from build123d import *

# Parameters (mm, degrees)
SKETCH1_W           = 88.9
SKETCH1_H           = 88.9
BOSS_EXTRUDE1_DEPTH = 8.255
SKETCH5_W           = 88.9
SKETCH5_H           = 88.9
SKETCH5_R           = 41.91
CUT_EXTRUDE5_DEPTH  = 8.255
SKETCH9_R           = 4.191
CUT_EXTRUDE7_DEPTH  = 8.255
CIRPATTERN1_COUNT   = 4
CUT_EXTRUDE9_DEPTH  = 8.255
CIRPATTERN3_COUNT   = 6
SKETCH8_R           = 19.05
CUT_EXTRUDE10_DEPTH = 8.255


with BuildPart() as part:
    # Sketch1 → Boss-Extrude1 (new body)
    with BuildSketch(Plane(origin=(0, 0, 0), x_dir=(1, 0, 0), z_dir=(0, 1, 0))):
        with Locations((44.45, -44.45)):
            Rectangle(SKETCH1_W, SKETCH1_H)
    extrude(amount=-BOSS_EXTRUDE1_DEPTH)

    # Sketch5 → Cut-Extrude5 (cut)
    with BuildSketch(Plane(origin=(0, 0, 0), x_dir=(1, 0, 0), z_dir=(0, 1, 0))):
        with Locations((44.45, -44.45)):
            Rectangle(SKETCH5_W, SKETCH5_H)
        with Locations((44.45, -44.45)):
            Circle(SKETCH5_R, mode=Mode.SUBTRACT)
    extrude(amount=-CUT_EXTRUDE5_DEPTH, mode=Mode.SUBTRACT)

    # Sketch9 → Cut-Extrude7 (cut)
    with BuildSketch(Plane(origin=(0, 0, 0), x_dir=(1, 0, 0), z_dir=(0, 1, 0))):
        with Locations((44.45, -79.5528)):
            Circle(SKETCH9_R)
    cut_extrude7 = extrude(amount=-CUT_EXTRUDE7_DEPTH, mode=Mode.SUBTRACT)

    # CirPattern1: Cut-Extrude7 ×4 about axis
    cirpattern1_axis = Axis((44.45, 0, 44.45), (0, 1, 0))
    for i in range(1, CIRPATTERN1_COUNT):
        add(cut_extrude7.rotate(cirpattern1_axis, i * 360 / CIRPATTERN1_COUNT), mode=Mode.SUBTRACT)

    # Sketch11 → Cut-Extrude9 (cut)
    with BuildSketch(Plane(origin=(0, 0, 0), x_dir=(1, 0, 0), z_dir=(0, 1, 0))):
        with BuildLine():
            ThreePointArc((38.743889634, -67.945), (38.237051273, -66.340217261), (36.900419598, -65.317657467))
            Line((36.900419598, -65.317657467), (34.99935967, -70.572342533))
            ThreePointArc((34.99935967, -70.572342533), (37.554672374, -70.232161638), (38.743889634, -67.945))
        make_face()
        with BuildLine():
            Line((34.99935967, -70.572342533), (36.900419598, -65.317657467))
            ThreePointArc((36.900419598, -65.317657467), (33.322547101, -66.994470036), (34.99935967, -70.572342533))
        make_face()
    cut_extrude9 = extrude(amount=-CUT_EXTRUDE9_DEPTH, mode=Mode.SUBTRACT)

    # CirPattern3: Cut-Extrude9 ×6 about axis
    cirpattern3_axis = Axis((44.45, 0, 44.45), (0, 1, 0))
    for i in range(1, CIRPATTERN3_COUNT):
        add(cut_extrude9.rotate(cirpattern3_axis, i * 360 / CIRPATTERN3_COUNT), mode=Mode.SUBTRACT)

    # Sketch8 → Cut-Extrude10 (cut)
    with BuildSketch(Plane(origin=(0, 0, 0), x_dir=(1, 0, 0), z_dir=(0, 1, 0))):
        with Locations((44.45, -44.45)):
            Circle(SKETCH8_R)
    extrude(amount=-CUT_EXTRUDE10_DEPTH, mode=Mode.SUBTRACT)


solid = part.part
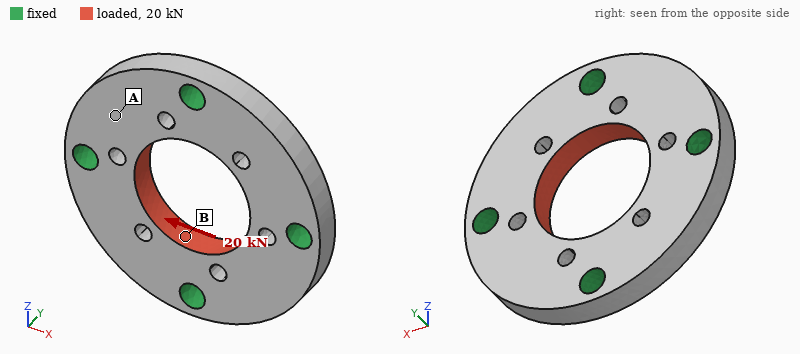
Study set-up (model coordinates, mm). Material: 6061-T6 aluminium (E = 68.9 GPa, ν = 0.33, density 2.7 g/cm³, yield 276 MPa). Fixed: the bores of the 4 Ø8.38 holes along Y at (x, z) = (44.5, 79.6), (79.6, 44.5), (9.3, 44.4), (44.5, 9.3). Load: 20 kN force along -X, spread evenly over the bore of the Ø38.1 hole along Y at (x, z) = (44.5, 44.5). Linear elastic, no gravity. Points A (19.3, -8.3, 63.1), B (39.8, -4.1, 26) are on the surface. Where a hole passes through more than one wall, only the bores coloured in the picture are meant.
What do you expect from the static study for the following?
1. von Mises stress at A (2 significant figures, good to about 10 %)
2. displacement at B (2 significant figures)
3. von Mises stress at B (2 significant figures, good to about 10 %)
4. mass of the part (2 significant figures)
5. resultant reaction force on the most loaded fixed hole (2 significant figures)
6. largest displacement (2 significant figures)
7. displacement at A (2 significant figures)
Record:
10.0 MPa
14 µm
35 MPa
89 g
5.3 kN
15 µm
10 µm
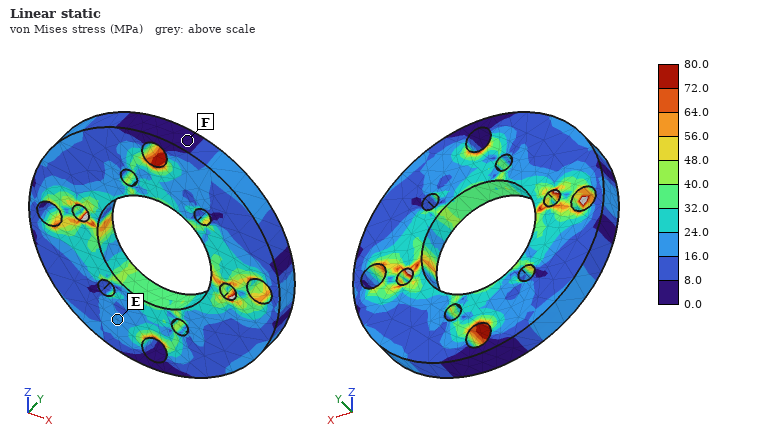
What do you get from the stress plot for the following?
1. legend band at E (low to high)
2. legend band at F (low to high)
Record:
16.0 to 24.0 MPa
0.0 to 8.0 MPa
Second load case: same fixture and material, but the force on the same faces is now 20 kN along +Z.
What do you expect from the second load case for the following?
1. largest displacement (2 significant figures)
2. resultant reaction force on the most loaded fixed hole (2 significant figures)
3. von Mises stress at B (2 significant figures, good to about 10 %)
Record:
15 µm
5.3 kN
29 MPa
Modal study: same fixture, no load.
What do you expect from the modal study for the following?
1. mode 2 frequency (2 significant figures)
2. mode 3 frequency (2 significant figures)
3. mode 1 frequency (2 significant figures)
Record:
14 kHz
14 kHz
14 kHz
